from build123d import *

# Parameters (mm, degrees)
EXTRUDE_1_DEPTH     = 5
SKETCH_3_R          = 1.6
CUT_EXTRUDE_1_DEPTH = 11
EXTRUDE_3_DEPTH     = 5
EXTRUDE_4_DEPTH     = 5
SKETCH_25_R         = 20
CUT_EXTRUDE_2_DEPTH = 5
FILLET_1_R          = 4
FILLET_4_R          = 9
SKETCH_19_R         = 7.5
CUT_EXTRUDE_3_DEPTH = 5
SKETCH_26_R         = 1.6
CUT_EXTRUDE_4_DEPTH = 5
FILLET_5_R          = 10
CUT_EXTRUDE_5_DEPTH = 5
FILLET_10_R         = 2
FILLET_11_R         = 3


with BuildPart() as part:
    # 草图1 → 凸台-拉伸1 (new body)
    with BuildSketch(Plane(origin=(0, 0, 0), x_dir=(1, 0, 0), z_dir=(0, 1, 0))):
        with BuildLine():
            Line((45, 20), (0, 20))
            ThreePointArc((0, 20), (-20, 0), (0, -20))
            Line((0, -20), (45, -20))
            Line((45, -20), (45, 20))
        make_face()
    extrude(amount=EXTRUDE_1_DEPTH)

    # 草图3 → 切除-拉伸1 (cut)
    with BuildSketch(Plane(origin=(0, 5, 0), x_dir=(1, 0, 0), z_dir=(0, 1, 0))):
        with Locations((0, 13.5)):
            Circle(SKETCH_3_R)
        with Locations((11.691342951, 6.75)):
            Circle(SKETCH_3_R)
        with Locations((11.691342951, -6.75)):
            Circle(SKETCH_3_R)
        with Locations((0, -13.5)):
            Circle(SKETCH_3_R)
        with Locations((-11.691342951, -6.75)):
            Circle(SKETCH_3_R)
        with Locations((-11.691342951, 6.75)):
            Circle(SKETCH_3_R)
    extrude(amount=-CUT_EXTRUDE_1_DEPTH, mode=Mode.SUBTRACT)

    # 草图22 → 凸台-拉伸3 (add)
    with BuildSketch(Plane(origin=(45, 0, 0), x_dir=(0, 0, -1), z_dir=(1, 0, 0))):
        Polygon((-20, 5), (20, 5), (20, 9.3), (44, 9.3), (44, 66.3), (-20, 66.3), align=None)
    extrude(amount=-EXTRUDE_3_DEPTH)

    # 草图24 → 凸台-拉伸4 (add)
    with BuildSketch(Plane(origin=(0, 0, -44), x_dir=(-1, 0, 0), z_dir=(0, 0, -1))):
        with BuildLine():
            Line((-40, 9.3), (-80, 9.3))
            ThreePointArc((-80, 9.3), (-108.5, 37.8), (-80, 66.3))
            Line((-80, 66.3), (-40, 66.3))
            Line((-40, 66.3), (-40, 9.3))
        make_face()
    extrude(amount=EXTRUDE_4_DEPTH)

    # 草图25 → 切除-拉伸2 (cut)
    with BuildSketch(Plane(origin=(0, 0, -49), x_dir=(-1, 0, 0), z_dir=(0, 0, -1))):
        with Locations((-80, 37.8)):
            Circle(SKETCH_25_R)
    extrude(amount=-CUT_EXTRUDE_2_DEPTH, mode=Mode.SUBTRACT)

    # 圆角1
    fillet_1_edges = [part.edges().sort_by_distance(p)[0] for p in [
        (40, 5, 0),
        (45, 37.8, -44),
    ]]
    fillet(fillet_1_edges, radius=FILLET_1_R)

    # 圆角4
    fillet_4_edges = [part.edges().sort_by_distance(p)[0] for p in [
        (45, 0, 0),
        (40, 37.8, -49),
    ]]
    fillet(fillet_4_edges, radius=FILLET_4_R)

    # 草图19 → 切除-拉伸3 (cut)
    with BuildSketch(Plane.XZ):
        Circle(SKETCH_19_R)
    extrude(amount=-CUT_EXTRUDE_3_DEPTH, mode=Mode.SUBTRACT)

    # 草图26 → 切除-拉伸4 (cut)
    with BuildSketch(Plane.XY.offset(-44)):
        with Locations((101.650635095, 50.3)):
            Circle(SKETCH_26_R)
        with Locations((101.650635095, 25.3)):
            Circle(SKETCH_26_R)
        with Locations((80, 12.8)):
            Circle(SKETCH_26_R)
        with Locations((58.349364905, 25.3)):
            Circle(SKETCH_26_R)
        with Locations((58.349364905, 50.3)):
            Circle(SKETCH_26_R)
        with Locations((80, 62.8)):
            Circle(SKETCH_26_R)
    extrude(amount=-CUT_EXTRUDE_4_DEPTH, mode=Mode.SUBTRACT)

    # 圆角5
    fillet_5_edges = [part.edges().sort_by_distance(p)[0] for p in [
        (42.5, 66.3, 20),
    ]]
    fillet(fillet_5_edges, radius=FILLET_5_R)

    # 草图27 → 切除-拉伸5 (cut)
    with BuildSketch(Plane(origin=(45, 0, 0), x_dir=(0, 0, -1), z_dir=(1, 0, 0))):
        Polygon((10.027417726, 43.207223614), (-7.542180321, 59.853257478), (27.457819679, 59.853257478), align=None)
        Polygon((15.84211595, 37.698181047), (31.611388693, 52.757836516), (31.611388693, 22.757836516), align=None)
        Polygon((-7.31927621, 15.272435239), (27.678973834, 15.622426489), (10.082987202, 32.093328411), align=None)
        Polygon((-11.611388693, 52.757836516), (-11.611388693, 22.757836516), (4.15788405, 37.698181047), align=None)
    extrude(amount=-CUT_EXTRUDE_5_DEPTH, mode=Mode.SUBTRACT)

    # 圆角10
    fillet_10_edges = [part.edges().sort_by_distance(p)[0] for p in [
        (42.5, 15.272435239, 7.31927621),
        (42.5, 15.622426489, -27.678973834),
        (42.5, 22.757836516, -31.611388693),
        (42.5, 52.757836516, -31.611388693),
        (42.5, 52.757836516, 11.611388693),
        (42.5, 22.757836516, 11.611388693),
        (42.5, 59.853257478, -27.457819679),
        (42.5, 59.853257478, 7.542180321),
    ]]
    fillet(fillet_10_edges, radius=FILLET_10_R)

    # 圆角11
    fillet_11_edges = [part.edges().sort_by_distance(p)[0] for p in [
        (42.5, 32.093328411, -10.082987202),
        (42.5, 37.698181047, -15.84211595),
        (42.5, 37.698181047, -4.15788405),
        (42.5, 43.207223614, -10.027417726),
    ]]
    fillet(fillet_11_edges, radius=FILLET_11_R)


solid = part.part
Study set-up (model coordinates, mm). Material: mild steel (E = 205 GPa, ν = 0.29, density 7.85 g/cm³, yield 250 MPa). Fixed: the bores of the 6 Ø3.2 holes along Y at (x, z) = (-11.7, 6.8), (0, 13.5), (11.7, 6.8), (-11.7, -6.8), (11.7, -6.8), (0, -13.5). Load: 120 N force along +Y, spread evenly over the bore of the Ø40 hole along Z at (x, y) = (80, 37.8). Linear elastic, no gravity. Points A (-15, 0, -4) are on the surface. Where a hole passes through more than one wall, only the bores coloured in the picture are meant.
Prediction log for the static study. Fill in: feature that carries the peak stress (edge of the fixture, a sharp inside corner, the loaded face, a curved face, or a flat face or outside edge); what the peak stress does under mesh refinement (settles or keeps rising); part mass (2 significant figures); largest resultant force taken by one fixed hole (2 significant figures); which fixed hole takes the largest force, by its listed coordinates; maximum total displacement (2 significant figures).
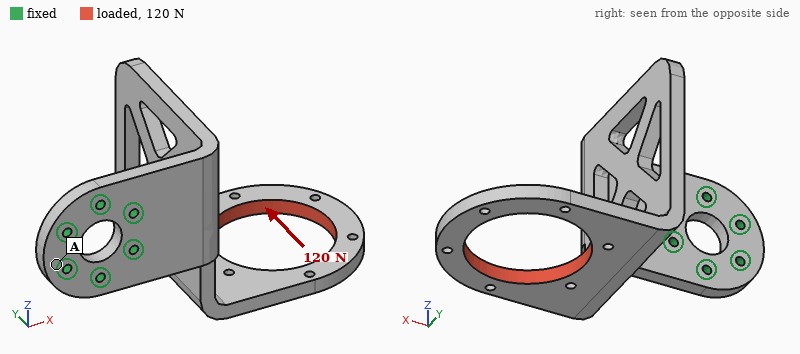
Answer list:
edge of the fixture
keeps rising
270 g
460 N
(11.7, -6.8)
0.49 mm
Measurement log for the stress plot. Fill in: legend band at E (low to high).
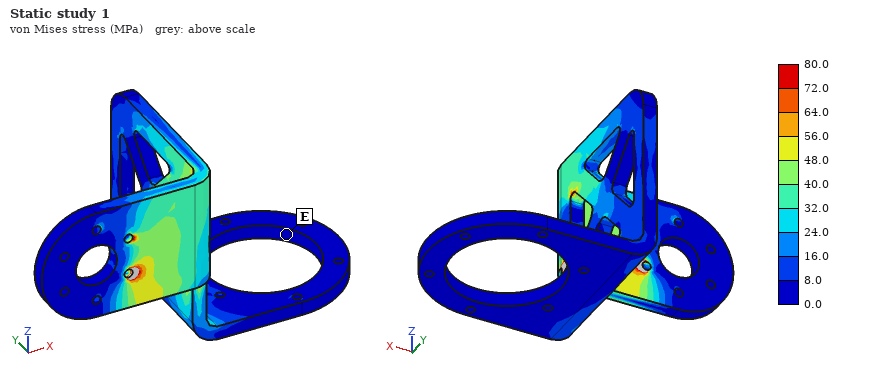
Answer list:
0.0 to 8.0 MPa
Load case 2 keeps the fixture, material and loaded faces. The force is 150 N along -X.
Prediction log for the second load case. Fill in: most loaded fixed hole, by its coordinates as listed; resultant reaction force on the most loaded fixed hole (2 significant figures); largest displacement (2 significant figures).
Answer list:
(11.7, -6.8)
250 N
0.48 mm
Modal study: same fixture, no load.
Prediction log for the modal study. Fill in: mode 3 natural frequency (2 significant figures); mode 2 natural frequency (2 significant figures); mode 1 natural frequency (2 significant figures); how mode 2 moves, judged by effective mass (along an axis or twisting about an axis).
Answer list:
670 Hz
460 Hz
260 Hz
along Z
